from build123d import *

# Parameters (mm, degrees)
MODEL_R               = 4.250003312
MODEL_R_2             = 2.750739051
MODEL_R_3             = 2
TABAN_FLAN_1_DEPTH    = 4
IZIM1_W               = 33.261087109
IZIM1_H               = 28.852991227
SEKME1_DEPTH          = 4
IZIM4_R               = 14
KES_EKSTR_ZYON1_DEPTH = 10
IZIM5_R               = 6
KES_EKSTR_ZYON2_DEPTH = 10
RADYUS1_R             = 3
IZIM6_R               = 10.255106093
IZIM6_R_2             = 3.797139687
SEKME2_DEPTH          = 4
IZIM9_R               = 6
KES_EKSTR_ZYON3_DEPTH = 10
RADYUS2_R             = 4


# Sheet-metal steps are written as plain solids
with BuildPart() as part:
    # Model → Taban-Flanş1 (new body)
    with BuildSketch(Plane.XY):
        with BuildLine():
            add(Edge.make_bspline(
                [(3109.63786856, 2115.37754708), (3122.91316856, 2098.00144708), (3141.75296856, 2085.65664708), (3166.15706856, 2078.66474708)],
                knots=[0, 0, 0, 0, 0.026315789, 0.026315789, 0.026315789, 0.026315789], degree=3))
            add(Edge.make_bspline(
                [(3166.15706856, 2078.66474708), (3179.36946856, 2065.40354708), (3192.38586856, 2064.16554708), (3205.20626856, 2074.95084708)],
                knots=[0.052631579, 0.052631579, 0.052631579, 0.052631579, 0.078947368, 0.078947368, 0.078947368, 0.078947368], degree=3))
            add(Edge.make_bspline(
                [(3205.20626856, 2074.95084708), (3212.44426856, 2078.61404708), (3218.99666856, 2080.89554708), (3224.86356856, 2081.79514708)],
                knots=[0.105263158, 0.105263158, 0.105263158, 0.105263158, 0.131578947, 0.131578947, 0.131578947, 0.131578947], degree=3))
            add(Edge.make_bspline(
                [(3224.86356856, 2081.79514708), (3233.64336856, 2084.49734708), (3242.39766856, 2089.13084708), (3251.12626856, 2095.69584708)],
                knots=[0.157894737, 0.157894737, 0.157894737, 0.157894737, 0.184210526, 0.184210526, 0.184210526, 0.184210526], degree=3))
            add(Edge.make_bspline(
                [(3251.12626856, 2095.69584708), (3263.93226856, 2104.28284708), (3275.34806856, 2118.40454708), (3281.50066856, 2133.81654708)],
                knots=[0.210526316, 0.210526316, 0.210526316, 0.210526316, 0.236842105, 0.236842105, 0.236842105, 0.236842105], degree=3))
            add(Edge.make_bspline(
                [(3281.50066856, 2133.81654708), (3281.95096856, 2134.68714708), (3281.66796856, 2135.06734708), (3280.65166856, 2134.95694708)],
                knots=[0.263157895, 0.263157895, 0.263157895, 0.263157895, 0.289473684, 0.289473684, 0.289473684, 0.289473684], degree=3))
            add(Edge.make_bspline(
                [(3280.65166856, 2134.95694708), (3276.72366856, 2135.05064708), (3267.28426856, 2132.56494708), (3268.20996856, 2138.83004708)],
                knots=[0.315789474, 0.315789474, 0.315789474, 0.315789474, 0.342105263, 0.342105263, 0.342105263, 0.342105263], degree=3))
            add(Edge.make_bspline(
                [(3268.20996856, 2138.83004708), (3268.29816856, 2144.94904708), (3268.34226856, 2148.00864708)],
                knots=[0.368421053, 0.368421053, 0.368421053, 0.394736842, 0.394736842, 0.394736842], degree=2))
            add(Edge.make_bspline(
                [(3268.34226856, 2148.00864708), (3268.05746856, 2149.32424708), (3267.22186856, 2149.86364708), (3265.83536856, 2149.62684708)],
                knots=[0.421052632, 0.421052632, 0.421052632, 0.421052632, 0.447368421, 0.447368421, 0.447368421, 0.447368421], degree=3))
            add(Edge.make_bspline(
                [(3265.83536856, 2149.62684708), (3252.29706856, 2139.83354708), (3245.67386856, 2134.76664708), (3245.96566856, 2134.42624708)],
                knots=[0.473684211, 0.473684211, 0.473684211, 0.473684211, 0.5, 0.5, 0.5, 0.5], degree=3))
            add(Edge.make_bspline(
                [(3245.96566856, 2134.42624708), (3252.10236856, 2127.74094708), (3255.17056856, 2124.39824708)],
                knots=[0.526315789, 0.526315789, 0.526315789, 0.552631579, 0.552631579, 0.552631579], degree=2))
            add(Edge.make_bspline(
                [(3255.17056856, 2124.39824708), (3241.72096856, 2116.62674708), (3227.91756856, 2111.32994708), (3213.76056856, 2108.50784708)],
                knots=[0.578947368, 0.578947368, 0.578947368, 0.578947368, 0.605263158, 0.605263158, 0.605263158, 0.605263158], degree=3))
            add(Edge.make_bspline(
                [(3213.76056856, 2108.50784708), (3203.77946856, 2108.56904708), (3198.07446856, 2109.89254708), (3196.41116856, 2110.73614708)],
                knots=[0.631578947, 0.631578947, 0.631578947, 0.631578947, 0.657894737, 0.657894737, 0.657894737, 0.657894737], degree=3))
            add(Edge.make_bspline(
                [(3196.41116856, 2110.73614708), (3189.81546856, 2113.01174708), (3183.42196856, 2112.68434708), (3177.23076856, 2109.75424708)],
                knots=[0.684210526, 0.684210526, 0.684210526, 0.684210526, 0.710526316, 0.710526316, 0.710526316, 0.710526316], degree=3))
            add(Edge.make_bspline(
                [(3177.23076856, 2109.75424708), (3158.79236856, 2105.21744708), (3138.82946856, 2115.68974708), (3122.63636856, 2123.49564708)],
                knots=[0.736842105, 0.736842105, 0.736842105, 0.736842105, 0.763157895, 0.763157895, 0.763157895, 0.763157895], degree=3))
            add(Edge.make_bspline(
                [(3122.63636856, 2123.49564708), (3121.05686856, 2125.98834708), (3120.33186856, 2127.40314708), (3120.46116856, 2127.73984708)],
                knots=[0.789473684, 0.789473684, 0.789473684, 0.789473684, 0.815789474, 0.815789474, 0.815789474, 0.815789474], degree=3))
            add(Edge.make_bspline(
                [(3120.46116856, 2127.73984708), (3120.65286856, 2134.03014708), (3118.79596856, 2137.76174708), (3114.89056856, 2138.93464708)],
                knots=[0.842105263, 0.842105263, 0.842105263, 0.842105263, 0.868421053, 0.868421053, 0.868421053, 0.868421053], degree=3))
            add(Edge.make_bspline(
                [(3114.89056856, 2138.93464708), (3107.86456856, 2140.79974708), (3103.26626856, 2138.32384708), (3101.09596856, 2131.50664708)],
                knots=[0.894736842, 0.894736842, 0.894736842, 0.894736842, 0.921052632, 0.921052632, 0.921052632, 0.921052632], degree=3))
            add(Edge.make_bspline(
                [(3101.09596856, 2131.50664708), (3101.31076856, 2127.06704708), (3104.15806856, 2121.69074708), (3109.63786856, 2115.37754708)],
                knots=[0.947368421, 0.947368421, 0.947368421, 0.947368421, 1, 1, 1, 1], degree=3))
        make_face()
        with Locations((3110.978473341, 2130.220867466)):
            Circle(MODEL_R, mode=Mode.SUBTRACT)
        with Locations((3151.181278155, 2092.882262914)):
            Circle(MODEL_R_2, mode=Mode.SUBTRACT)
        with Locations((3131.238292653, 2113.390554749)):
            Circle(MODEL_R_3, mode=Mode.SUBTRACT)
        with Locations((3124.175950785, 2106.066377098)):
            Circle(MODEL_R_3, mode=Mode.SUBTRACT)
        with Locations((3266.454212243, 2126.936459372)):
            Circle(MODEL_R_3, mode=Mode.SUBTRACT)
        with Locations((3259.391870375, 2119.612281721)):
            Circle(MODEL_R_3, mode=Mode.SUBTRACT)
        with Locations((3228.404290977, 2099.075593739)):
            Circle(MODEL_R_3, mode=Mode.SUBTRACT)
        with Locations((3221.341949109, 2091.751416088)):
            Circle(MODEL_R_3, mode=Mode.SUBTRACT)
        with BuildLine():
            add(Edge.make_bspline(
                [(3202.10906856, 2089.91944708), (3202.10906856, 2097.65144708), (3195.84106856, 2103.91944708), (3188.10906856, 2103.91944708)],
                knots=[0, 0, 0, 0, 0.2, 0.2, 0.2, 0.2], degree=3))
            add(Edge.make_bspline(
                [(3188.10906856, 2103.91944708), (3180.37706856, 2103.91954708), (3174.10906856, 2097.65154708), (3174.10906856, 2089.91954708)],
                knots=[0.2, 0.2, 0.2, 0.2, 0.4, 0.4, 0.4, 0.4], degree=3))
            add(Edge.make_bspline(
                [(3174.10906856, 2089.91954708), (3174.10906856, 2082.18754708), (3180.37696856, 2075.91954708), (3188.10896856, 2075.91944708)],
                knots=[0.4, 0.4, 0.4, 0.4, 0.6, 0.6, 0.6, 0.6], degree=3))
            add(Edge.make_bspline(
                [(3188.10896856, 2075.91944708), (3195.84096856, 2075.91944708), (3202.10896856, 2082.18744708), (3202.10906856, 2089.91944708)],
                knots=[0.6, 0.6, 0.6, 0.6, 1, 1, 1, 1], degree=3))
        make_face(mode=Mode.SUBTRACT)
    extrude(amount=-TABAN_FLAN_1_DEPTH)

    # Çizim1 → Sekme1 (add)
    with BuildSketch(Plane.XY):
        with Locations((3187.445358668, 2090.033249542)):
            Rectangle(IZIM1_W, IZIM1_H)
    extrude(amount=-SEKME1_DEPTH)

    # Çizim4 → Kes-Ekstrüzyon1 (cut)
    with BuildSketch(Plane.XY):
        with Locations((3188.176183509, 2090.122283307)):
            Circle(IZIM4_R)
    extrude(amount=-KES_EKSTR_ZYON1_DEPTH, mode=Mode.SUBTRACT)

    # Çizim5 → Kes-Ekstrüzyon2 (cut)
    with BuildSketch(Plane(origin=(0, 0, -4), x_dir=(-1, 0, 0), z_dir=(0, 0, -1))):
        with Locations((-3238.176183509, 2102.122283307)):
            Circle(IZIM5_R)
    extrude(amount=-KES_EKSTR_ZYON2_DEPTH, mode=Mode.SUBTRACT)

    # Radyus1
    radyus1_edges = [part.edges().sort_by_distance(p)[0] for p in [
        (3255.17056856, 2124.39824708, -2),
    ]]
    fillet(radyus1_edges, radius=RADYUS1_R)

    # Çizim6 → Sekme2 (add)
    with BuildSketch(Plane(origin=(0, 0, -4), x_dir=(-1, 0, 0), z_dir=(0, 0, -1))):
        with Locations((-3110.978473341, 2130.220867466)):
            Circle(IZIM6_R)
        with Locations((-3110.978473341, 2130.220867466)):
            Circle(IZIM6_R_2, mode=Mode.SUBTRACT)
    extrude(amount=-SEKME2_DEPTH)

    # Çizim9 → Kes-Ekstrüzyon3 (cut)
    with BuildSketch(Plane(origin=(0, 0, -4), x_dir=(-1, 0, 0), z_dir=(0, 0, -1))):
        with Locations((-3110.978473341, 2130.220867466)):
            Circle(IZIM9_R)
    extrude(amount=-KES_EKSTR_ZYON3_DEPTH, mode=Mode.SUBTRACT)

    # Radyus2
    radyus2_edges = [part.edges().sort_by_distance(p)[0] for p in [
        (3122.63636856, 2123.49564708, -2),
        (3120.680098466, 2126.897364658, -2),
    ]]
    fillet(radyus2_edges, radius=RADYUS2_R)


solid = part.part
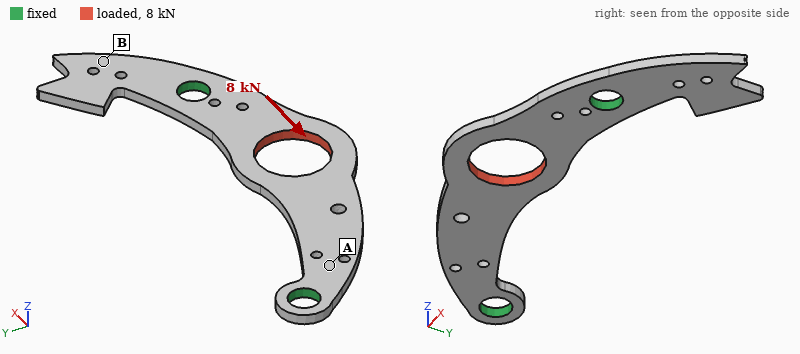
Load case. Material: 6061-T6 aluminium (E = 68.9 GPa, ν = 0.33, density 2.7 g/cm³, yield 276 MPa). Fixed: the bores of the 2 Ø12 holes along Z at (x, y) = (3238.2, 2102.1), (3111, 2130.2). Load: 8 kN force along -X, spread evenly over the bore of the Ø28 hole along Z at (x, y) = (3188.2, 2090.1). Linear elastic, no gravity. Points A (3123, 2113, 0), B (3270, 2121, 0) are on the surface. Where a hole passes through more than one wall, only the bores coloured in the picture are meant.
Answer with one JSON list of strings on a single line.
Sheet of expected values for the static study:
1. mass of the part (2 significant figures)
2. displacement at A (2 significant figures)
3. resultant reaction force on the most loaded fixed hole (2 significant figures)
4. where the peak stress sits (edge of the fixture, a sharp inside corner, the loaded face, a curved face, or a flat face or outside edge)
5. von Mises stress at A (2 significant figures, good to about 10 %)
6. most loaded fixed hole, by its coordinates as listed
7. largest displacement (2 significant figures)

["49 g", "30 µm", "6.1 kN", "a curved face", "39 MPa", "(3238.2, 2102.1)", "99 µm"]
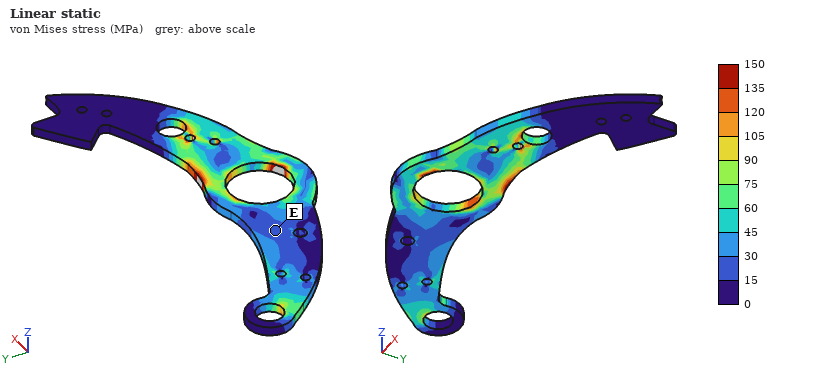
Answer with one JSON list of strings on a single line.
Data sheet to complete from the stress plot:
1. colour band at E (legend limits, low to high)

["15 to 30 MPa"]
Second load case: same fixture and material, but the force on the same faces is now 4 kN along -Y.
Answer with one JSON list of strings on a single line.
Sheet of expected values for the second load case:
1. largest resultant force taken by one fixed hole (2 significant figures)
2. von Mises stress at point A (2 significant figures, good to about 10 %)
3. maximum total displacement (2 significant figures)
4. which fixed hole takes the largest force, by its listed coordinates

["2.9 kN", "37 MPa", "0.14 mm", "(3238.2, 2102.1)"]
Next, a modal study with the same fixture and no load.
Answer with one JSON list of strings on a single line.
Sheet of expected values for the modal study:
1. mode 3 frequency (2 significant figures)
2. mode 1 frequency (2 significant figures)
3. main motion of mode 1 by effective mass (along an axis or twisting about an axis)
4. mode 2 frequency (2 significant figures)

["2500 Hz", "980 Hz", "along Z", "1400 Hz"]
